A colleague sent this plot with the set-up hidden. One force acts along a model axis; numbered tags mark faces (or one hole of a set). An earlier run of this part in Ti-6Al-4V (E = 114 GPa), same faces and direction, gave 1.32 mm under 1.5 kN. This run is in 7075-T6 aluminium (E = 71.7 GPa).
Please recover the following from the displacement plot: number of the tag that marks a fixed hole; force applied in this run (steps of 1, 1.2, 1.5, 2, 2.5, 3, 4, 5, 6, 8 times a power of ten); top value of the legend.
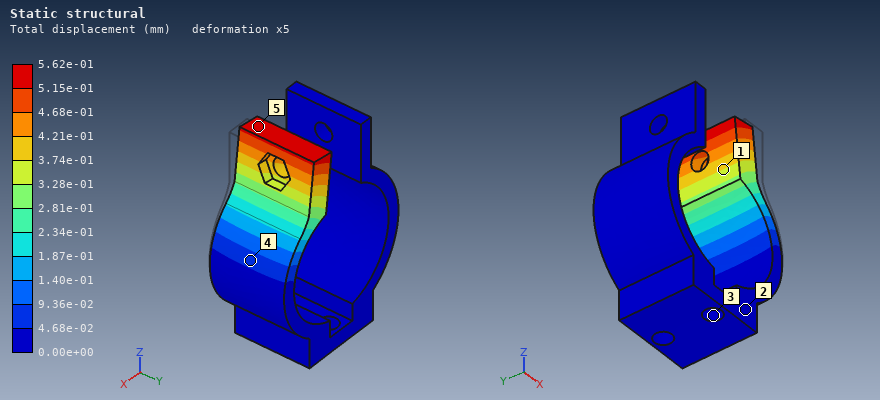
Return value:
3
400 N
5.62e-01 mm
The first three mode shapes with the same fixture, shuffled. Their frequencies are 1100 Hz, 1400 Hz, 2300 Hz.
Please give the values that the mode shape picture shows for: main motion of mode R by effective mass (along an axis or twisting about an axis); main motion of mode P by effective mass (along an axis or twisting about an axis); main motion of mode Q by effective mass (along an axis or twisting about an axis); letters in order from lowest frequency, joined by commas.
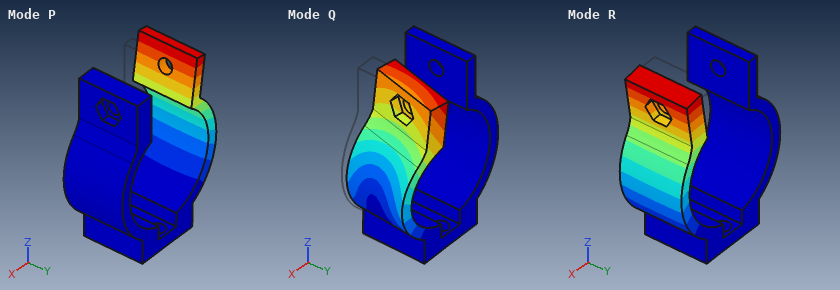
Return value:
along X
along X
along Y
R, P, Q
